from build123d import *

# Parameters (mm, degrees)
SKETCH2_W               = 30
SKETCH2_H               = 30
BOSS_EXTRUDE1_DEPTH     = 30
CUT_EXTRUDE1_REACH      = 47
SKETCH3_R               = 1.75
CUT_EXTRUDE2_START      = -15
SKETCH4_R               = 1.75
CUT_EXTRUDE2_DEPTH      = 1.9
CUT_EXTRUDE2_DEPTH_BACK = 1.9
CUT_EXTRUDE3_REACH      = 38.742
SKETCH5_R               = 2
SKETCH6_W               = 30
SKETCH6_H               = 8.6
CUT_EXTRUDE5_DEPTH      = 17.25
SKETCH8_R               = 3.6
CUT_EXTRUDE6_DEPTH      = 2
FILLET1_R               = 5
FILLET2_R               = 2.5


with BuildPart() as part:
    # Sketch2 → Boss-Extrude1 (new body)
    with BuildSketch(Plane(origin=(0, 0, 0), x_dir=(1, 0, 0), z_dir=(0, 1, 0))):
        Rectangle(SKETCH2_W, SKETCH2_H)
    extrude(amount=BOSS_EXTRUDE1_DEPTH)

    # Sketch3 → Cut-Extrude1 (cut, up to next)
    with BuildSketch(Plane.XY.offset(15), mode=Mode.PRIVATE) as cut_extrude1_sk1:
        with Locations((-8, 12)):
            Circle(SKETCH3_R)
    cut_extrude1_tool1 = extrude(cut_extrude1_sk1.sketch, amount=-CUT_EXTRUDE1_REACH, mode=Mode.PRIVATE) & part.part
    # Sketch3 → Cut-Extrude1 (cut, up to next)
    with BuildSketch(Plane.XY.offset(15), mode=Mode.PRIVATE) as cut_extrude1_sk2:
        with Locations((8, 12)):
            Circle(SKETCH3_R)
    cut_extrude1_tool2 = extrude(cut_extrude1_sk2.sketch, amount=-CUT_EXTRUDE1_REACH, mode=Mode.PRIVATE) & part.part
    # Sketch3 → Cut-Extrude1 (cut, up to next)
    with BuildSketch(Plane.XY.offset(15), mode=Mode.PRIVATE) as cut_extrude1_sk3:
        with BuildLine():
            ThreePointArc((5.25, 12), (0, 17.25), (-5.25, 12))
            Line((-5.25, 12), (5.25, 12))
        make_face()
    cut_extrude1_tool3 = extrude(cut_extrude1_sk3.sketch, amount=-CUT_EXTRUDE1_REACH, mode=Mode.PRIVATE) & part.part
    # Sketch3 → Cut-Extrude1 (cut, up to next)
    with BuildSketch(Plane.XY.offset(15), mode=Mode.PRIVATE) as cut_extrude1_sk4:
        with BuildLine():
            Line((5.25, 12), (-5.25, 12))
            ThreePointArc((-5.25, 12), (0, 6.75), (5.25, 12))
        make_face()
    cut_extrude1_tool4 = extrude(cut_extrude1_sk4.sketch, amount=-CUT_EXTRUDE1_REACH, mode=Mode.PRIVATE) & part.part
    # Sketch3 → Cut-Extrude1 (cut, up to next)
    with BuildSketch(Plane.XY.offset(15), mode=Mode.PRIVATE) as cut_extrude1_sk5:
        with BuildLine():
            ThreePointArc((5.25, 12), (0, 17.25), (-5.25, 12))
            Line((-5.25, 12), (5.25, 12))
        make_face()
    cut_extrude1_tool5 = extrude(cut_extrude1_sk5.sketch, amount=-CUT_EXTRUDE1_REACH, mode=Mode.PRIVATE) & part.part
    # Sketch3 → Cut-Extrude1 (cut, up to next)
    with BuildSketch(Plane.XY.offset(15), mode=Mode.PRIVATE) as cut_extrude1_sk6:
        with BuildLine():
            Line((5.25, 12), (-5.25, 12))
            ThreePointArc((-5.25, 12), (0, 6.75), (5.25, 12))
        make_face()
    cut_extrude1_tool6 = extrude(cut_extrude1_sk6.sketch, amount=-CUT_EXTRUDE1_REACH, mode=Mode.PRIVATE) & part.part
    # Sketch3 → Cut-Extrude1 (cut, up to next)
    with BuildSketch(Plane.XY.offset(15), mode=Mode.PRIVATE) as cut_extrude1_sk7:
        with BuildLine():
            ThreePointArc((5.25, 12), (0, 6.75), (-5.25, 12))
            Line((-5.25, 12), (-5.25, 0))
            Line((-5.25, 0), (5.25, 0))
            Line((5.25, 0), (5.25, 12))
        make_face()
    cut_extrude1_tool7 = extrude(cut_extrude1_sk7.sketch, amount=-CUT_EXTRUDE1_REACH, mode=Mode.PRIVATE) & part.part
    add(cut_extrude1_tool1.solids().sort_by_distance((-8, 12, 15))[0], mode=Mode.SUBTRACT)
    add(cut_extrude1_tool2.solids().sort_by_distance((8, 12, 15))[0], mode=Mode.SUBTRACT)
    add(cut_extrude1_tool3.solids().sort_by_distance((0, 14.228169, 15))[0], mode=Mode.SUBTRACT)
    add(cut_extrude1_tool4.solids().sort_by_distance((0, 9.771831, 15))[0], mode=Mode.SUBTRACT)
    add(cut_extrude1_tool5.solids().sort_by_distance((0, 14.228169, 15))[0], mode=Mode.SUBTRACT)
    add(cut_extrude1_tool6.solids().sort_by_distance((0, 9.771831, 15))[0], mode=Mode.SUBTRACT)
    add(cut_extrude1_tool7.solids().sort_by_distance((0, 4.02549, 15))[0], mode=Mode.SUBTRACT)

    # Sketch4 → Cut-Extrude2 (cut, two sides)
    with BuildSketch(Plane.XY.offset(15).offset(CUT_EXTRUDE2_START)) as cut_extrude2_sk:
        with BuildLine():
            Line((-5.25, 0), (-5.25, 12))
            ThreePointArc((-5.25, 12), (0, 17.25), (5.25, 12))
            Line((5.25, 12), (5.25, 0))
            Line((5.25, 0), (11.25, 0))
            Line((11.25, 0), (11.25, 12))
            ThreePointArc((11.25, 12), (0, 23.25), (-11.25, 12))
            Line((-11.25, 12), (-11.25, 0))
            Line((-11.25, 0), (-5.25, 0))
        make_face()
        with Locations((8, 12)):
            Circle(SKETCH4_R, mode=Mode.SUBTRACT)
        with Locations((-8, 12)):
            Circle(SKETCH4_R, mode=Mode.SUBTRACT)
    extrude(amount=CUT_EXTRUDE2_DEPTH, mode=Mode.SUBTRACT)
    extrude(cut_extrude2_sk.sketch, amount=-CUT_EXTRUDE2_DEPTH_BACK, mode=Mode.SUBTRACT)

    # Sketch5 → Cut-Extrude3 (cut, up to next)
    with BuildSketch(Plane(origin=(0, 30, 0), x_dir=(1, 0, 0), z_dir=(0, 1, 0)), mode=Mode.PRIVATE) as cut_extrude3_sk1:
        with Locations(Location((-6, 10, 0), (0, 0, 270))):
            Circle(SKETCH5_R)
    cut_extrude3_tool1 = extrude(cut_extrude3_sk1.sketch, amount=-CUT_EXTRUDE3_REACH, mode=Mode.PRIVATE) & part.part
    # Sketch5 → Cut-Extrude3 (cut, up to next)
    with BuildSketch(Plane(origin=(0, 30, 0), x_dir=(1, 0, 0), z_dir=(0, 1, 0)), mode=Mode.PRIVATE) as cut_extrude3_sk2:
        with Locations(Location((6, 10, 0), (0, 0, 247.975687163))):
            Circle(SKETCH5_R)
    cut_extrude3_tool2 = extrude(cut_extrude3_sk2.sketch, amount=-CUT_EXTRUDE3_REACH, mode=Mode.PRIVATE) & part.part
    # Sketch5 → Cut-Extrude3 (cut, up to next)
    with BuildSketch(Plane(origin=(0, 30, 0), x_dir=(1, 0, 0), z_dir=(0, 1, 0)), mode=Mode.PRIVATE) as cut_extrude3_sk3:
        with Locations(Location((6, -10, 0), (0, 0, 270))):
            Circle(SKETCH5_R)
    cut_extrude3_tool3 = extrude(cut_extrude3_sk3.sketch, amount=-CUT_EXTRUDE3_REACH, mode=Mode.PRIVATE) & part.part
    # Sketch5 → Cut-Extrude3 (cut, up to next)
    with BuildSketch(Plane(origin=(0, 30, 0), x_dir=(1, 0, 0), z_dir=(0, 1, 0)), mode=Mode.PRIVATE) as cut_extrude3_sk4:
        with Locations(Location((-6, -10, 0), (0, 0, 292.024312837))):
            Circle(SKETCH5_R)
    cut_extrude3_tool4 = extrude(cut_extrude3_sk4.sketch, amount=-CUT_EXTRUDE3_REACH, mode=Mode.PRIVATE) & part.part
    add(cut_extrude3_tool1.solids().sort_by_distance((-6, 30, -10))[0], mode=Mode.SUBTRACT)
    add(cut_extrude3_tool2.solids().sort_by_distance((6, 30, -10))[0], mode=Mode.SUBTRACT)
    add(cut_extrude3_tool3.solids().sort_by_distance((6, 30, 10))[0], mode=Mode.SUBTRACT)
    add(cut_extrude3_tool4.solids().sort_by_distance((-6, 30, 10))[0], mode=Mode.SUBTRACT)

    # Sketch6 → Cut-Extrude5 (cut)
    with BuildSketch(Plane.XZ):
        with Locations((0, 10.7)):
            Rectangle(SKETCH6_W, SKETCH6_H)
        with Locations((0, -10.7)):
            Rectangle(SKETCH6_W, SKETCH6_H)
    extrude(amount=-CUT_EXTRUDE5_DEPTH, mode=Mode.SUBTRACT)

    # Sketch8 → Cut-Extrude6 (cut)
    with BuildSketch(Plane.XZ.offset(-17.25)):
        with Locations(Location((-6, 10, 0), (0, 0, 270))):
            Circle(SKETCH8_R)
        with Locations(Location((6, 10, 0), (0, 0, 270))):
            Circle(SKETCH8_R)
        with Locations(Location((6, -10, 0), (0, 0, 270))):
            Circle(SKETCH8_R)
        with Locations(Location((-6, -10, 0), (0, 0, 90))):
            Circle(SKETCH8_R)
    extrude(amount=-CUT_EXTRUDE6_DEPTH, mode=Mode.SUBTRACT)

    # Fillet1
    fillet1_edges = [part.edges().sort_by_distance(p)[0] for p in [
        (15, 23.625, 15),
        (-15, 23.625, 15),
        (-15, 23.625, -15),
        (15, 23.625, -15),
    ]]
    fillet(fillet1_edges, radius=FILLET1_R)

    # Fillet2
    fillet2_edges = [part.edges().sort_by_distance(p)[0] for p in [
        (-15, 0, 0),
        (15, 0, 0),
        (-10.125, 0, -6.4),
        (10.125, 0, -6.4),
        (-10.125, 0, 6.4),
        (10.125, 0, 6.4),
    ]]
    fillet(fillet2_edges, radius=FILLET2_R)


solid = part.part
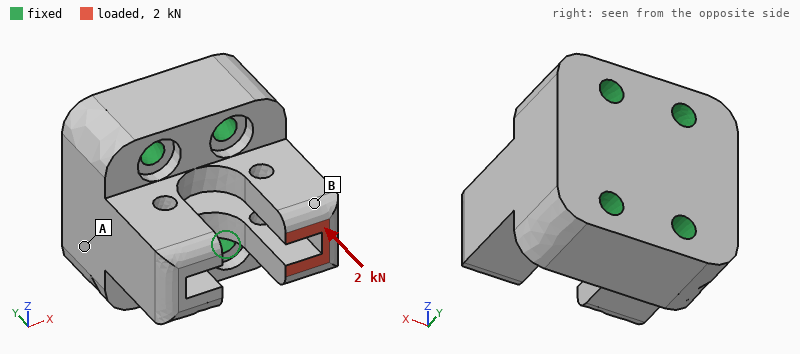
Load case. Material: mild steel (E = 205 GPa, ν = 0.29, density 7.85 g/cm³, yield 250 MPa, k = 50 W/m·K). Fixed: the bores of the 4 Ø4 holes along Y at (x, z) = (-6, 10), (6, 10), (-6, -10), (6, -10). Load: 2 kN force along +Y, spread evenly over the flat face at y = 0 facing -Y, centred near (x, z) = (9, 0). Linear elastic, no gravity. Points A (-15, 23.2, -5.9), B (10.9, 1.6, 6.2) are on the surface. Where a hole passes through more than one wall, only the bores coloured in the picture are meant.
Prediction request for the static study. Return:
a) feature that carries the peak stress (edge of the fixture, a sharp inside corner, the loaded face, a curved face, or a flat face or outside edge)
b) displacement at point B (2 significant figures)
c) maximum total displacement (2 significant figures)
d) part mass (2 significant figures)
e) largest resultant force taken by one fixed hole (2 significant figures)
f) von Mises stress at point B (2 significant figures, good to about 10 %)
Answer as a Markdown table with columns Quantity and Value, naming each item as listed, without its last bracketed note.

| Quantity | Value |
|---|---|
| feature that carries the peak stress | a curved face |
| displacement at point B | 2.7 µm |
| maximum total displacement | 6.0 µm |
| part mass | 110 g |
| largest resultant force taken by one fixed hole | 970 N |
| von Mises stress at point B | 17 MPa |
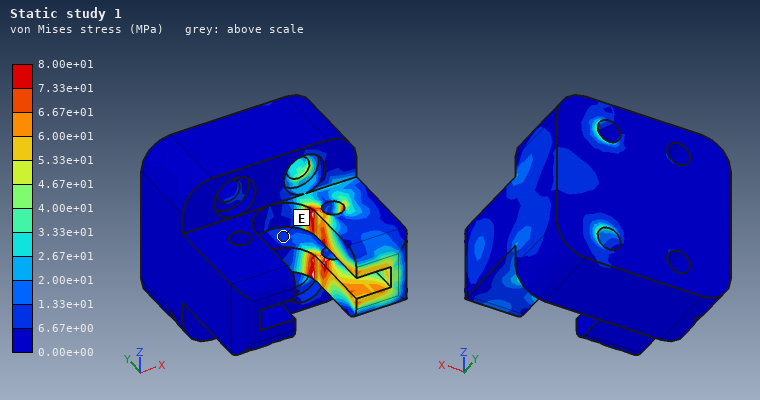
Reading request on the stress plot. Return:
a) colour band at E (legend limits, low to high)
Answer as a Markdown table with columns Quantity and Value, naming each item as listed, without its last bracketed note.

| Quantity | Value |
|---|---|
| colour band at E | 6.67e+00 to 1.33e+01 MPa |
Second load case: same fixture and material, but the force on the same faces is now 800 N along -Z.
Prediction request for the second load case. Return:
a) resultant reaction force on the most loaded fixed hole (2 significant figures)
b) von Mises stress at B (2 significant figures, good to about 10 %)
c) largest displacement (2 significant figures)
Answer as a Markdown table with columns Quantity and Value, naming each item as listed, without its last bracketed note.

| Quantity | Value |
|---|---|
| resultant reaction force on the most loaded fixed hole | 980 N |
| von Mises stress at B | 39 MPa |
| largest displacement | 24 µm |
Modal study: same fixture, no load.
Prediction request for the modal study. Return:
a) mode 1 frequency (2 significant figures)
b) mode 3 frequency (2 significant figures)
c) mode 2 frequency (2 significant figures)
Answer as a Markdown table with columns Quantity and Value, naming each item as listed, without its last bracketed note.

| Quantity | Value |
|---|---|
| mode 1 frequency | 16 kHz |
| mode 3 frequency | 17 kHz |
| mode 2 frequency | 16 kHz |
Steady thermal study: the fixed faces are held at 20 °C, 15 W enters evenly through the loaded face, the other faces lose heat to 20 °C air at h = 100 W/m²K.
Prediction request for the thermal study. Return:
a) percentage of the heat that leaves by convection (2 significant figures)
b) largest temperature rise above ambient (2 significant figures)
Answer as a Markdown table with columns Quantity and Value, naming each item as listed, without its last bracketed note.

| Quantity | Value |
|---|---|
| percentage of the heat that leaves by convection | 26 % |
| largest temperature rise above ambient | 69 K |
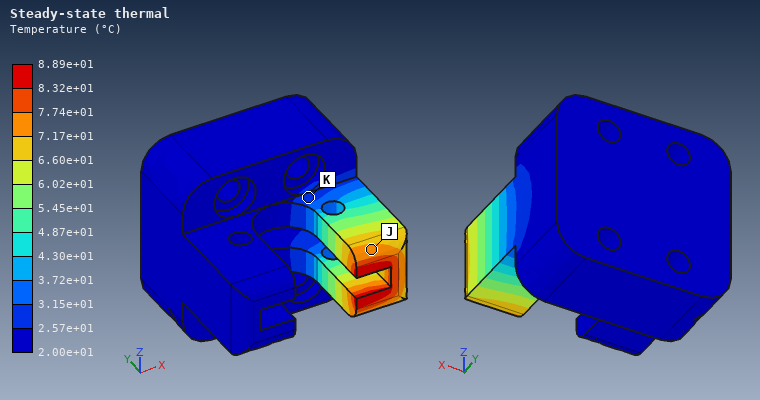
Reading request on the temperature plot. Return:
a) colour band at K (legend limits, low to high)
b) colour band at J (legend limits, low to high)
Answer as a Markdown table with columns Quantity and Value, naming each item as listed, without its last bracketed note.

| Quantity | Value |
|---|---|
| colour band at K | 2.57e+01 to 3.15e+01 °C |
| colour band at J | 7.17e+01 to 7.74e+01 °C |
